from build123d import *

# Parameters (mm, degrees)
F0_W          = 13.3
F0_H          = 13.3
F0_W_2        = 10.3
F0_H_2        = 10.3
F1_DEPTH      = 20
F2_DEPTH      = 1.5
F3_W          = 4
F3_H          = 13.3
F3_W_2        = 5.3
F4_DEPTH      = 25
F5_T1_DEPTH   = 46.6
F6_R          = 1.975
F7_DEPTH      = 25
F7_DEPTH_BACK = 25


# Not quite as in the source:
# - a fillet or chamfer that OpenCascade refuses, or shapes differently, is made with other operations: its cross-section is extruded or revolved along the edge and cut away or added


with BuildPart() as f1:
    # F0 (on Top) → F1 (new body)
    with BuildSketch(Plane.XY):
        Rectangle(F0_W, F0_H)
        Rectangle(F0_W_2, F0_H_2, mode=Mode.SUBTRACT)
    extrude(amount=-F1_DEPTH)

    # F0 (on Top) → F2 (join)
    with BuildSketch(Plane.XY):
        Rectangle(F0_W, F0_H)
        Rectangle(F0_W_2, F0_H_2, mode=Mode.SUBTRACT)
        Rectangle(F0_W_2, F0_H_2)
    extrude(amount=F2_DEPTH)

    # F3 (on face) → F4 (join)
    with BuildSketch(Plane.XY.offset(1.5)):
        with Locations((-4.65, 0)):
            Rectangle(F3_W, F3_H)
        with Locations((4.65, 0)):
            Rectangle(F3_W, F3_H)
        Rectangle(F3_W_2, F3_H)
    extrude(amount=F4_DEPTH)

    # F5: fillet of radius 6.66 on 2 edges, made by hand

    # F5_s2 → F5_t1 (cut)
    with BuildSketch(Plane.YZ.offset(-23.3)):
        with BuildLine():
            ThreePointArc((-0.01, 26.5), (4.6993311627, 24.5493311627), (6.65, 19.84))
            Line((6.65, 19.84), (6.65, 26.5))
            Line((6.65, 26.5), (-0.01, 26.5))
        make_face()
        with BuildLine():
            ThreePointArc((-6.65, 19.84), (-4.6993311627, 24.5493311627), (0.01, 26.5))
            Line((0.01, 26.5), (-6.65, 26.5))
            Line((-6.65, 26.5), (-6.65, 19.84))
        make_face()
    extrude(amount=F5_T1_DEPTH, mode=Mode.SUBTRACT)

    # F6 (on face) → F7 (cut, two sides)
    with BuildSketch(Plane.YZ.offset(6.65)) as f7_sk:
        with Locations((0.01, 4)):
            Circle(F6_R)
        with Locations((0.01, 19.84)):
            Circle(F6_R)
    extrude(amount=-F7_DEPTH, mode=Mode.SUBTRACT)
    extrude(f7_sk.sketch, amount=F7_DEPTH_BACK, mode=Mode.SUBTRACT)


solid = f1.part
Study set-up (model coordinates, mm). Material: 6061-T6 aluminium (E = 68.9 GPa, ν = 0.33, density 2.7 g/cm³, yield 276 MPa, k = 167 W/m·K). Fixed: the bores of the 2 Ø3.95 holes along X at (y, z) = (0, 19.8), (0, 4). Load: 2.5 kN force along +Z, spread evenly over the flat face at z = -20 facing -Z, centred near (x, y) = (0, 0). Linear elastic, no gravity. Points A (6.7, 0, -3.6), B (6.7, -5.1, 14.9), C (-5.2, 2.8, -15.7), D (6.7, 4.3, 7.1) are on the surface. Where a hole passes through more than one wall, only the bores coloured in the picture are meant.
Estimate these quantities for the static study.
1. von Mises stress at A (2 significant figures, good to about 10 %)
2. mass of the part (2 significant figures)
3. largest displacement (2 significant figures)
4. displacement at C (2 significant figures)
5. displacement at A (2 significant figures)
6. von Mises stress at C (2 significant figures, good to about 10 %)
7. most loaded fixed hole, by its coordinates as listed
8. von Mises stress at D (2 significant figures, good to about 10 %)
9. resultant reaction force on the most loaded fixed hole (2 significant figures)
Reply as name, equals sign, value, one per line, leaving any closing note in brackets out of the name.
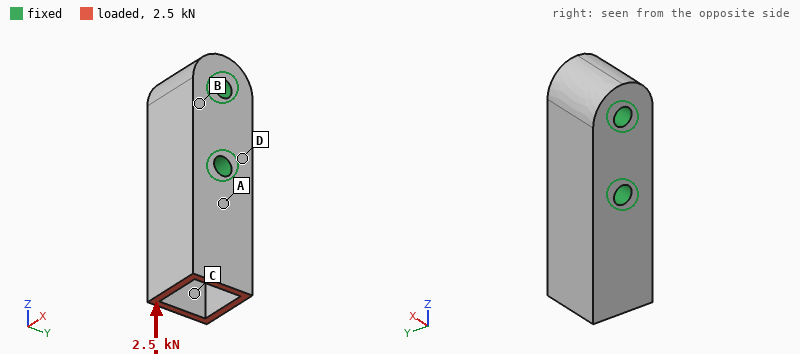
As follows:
von Mises stress at A = 42 MPa
mass of the part = 15 g
largest displacement = 13 µm
displacement at C = 10 µm
displacement at A = 3.9 µm
von Mises stress at C = 36 MPa
most loaded fixed hole, by its coordinates as listed = (0, 4)
von Mises stress at D = 10.0 MPa
resultant reaction force on the most loaded fixed hole = 2.1 kN
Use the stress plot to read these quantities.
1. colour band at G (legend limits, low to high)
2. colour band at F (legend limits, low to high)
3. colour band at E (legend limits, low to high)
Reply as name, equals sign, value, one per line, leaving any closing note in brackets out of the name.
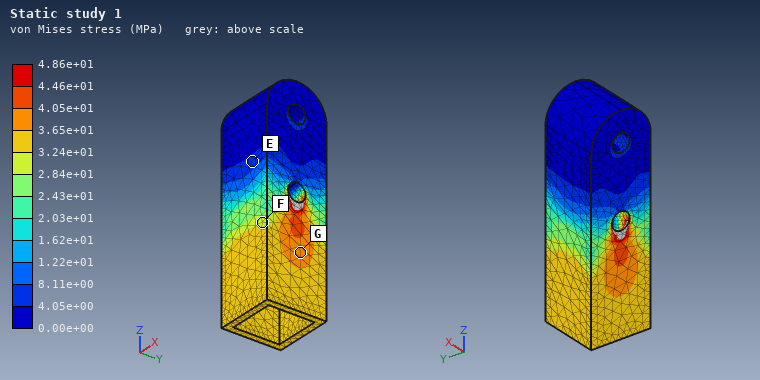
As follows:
colour band at G = 3.65e+01 to 4.05e+01 MPa
colour band at F = 2.84e+01 to 3.24e+01 MPa
colour band at E = 4.05e+00 to 8.11e+00 MPa
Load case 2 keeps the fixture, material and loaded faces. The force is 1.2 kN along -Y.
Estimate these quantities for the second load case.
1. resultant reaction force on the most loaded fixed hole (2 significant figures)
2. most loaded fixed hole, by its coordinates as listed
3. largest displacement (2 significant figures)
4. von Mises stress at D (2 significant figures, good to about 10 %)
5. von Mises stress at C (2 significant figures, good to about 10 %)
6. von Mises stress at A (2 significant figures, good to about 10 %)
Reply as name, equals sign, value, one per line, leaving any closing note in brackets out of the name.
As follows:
resultant reaction force on the most loaded fixed hole = 2.2 kN
most loaded fixed hole, by its coordinates as listed = (0, 4)
largest displacement = 0.13 mm
von Mises stress at D = 28 MPa
von Mises stress at C = 68 MPa
von Mises stress at A = 68 MPa
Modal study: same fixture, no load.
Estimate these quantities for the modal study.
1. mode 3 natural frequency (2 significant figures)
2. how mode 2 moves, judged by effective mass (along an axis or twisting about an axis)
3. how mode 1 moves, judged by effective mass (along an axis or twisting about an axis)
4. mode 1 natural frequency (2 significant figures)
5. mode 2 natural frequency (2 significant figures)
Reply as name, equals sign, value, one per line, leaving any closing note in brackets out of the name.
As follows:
mode 3 natural frequency = 20 kHz
how mode 2 moves, judged by effective mass = along X
how mode 1 moves, judged by effective mass = along Y
mode 1 natural frequency = 15 kHz
mode 2 natural frequency = 16 kHz
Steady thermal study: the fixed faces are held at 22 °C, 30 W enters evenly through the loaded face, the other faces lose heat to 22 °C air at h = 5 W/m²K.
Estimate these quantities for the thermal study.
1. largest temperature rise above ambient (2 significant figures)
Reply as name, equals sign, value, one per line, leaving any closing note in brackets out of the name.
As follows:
largest temperature rise above ambient = 57 K
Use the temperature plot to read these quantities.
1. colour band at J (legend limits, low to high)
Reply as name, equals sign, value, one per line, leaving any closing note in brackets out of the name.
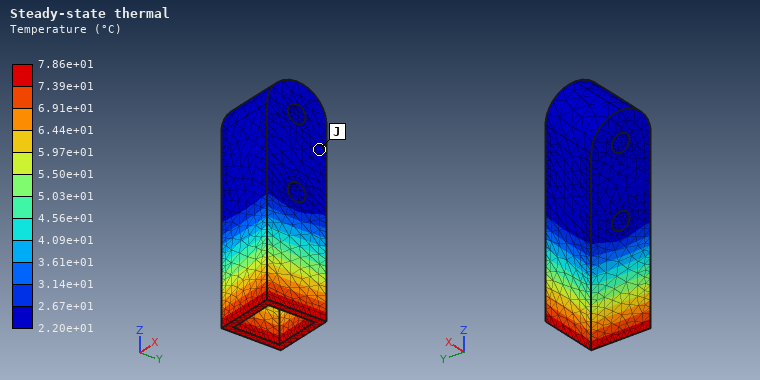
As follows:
colour band at J = 2.20e+01 to 2.67e+01 °C
